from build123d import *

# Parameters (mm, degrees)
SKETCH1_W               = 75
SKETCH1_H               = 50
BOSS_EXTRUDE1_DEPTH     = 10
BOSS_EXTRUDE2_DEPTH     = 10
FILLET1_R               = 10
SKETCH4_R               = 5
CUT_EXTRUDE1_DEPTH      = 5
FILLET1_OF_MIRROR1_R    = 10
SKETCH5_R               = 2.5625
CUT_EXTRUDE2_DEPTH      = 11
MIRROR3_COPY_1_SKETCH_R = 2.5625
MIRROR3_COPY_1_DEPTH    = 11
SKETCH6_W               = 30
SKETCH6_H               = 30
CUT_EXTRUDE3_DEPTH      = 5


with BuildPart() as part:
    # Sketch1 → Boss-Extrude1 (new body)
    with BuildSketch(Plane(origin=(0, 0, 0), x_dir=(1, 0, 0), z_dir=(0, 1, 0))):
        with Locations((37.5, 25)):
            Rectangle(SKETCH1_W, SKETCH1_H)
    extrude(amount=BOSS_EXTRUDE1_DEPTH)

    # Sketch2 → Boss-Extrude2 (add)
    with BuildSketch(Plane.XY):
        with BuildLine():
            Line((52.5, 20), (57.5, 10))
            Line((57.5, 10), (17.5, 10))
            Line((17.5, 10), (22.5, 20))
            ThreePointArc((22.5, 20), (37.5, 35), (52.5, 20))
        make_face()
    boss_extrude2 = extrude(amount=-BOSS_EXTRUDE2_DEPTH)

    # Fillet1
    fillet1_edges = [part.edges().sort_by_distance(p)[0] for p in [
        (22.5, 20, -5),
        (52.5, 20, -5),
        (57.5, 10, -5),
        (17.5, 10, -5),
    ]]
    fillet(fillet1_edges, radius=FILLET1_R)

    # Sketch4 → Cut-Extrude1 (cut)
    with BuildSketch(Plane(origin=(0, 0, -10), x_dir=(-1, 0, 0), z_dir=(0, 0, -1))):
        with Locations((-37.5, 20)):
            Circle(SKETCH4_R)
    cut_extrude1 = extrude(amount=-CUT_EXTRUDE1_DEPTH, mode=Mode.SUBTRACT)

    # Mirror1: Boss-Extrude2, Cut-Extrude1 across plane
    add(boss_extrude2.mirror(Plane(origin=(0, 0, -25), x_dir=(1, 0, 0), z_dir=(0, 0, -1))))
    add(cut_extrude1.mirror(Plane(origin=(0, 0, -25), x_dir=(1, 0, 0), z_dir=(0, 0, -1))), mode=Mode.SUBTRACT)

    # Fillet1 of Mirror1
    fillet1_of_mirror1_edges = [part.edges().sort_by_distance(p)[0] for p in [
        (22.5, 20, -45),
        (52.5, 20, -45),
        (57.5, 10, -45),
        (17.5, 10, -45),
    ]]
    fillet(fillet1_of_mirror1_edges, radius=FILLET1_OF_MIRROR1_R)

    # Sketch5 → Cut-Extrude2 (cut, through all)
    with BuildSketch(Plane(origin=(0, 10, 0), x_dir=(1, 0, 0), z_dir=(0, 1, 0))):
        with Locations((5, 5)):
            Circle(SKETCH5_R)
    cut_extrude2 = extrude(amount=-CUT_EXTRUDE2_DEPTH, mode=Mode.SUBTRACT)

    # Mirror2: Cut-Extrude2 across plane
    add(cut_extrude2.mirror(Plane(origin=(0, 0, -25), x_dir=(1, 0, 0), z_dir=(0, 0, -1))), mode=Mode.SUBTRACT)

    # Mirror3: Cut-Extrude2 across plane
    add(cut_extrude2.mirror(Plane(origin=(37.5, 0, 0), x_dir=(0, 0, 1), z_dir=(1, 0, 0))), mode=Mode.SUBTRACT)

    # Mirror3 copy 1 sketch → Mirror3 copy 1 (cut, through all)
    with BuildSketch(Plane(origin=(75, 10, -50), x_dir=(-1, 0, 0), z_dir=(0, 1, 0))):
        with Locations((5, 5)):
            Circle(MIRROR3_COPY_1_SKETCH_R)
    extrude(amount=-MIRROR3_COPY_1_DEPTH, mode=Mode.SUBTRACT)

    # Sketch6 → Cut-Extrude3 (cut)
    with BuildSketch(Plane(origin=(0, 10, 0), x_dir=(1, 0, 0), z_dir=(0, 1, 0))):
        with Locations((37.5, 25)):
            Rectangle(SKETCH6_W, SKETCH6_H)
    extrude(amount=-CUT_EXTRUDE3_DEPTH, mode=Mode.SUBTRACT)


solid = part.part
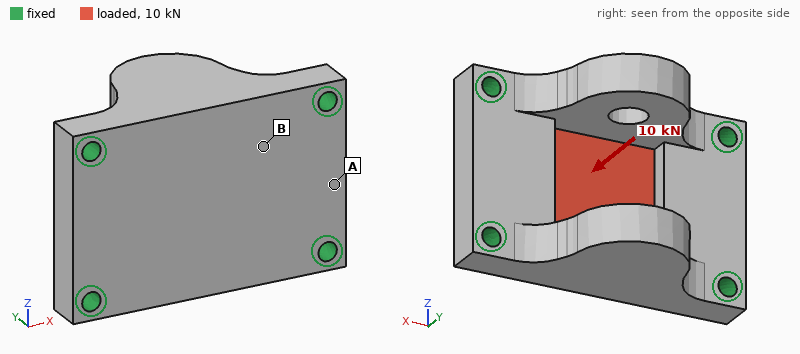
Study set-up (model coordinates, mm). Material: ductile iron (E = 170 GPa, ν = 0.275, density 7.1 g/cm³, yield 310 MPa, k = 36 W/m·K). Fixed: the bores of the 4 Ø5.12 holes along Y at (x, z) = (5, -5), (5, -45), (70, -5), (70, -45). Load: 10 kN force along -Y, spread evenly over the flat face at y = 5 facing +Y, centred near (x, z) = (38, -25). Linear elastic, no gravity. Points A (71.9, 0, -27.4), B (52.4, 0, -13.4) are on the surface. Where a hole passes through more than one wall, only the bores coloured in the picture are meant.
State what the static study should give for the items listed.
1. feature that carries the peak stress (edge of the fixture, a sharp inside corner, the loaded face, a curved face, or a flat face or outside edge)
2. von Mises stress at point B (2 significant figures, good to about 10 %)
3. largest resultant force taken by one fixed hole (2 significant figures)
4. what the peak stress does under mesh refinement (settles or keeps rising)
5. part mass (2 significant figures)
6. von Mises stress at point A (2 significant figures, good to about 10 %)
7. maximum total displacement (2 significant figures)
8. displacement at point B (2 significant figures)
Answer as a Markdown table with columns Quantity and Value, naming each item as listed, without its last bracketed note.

| Quantity | Value |
|---|---|
| feature that carries the peak stress | edge of the fixture |
| von Mises stress at point B | 43 MPa |
| largest resultant force taken by one fixed hole | 2.5 kN |
| what the peak stress does under mesh refinement | keeps rising |
| part mass | 320 g |
| von Mises stress at point A | 15 MPa |
| maximum total displacement | 36 µm |
| displacement at point B | 16 µm |
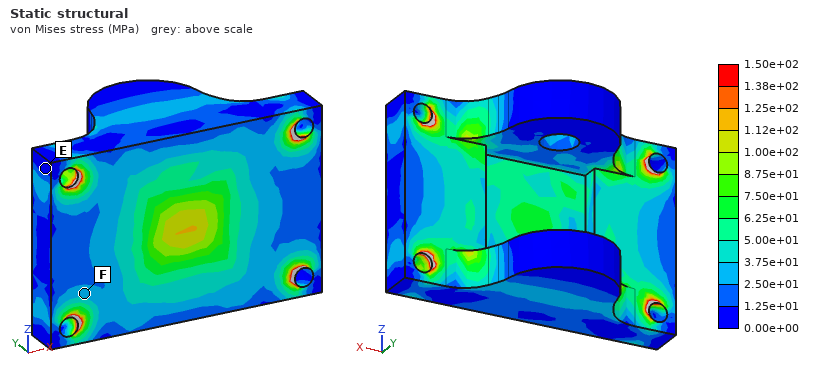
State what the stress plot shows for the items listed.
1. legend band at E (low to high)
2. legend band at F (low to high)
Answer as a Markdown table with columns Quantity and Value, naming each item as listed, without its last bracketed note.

| Quantity | Value |
|---|---|
| legend band at E | 0.00e+00 to 1.25e+01 MPa |
| legend band at F | 2.50e+01 to 3.75e+01 MPa |
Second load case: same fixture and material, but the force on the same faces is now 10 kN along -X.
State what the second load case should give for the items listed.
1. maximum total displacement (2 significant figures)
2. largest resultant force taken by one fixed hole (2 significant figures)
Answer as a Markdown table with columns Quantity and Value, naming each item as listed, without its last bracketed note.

| Quantity | Value |
|---|---|
| maximum total displacement | 4.8 µm |
| largest resultant force taken by one fixed hole | 2.6 kN |
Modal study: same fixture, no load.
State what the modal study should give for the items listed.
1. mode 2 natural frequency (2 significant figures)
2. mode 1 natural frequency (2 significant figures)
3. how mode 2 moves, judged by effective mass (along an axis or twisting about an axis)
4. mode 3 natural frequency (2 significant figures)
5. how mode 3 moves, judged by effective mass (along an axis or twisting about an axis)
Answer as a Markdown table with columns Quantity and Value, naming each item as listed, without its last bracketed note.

| Quantity | Value |
|---|---|
| mode 2 natural frequency | 6700 Hz |
| mode 1 natural frequency | 6300 Hz |
| how mode 2 moves, judged by effective mass | along Z |
| mode 3 natural frequency | 10 kHz |
| how mode 3 moves, judged by effective mass | along Y |
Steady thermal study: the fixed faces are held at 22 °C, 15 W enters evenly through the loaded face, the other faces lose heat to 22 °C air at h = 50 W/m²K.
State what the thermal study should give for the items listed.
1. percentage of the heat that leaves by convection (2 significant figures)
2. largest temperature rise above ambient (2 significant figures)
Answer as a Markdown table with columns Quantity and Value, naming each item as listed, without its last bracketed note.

| Quantity | Value |
|---|---|
| percentage of the heat that leaves by convection | 24 % |
| largest temperature rise above ambient | 16 K |
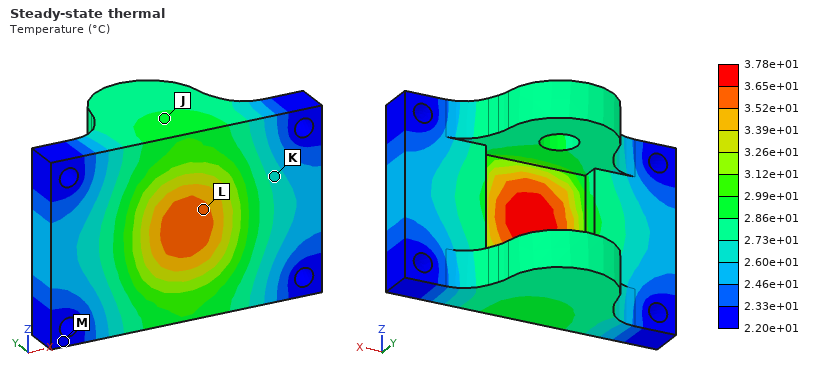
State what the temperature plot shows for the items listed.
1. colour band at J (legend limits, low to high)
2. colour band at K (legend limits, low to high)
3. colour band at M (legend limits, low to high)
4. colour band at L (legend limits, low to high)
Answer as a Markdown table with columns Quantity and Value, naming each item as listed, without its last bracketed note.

| Quantity | Value |
|---|---|
| colour band at J | 2.86e+01 to 2.99e+01 °C |
| colour band at K | 2.60e+01 to 2.73e+01 °C |
| colour band at M | 2.20e+01 to 2.33e+01 °C |
| colour band at L | 3.52e+01 to 3.65e+01 °C |
